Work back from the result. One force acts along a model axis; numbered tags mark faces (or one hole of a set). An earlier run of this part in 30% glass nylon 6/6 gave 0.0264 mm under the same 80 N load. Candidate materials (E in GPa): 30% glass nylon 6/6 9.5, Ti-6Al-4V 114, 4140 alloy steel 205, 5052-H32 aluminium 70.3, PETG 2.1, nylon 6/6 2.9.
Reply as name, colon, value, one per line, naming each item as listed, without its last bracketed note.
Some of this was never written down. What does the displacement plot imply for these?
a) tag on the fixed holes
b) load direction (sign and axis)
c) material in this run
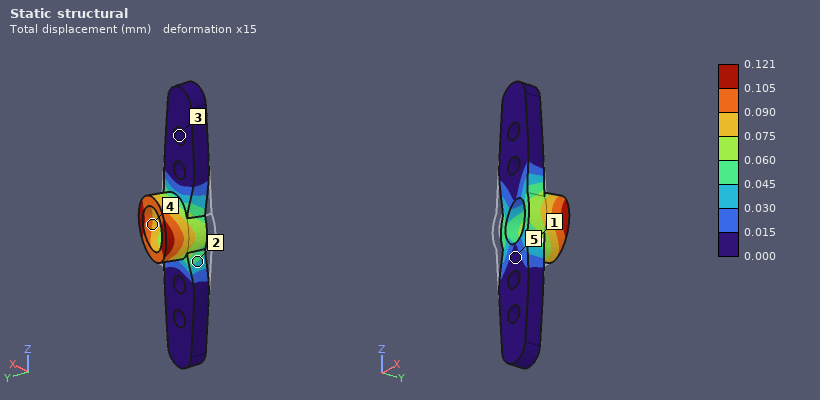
tag on the fixed holes: 3
load direction: +X
material in this run: PETG
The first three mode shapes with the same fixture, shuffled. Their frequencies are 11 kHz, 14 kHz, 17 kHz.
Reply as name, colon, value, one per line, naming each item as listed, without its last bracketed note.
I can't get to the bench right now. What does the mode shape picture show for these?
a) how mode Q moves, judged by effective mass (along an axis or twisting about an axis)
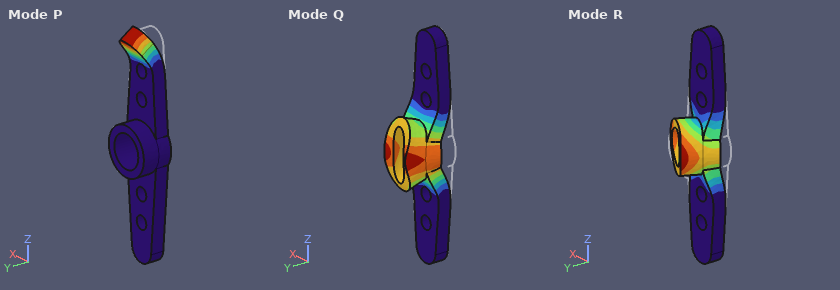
how mode Q moves, judged by effective mass: along Y
